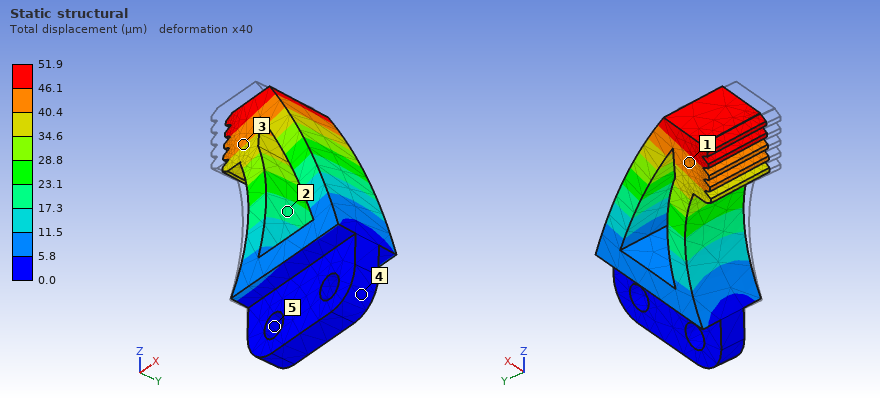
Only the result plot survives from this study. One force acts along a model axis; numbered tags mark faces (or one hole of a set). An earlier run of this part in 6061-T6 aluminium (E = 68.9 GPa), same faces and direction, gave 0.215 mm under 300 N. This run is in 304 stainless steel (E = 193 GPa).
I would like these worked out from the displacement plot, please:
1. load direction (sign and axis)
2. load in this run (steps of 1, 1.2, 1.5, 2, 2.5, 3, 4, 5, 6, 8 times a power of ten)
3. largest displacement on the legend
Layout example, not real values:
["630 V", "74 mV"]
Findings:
["+Y", "200 N", "51.9 µm"]
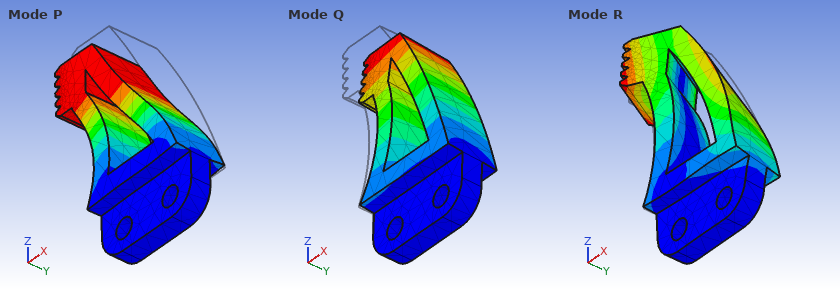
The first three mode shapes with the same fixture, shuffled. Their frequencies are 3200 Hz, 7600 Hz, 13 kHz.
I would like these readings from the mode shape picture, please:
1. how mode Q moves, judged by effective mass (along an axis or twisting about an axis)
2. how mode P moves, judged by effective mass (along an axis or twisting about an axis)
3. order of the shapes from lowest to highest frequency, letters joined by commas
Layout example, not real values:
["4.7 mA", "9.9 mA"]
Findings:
["along Y", "along X", "Q, P, R"]
